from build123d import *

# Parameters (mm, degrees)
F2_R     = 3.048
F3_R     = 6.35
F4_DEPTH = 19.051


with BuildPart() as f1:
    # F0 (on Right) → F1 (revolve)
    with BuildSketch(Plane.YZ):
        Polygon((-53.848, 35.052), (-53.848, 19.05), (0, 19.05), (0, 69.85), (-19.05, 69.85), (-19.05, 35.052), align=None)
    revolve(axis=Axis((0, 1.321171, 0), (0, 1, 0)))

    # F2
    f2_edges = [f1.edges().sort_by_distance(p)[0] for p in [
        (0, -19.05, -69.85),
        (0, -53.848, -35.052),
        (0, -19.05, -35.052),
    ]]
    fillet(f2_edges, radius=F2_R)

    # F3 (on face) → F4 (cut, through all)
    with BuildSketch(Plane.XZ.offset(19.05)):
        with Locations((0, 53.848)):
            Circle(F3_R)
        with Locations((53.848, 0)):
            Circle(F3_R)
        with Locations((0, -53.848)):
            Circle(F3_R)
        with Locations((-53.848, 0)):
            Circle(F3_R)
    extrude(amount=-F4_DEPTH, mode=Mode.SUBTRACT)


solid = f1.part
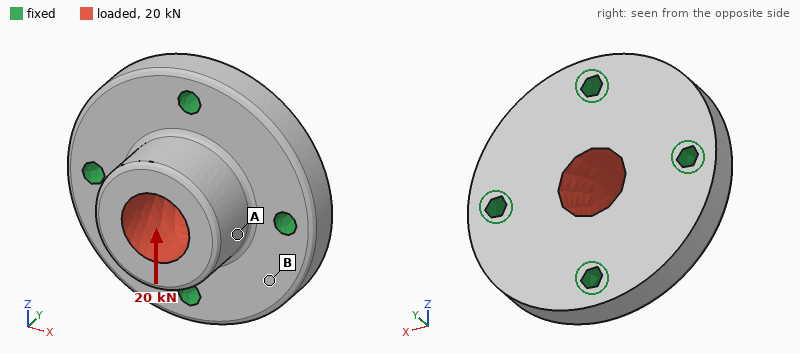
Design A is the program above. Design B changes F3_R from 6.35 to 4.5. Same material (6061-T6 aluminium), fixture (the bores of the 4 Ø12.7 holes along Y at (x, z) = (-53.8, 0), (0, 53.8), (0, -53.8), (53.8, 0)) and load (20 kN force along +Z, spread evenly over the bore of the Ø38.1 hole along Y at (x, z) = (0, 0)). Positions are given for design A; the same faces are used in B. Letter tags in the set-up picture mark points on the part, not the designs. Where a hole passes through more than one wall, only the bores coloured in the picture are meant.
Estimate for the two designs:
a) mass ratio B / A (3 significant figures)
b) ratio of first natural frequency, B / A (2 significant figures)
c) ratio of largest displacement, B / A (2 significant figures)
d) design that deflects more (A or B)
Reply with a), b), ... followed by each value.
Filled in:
a) 1.01
b) 0.92
c) 1.1
d) B
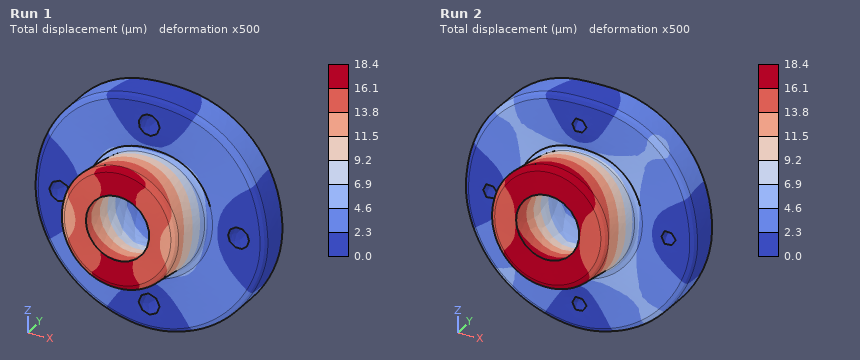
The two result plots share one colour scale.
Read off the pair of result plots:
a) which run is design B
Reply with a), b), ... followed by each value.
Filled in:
a) Run 2
